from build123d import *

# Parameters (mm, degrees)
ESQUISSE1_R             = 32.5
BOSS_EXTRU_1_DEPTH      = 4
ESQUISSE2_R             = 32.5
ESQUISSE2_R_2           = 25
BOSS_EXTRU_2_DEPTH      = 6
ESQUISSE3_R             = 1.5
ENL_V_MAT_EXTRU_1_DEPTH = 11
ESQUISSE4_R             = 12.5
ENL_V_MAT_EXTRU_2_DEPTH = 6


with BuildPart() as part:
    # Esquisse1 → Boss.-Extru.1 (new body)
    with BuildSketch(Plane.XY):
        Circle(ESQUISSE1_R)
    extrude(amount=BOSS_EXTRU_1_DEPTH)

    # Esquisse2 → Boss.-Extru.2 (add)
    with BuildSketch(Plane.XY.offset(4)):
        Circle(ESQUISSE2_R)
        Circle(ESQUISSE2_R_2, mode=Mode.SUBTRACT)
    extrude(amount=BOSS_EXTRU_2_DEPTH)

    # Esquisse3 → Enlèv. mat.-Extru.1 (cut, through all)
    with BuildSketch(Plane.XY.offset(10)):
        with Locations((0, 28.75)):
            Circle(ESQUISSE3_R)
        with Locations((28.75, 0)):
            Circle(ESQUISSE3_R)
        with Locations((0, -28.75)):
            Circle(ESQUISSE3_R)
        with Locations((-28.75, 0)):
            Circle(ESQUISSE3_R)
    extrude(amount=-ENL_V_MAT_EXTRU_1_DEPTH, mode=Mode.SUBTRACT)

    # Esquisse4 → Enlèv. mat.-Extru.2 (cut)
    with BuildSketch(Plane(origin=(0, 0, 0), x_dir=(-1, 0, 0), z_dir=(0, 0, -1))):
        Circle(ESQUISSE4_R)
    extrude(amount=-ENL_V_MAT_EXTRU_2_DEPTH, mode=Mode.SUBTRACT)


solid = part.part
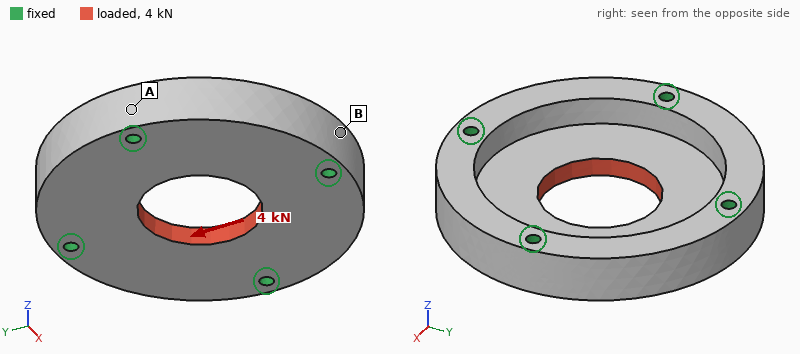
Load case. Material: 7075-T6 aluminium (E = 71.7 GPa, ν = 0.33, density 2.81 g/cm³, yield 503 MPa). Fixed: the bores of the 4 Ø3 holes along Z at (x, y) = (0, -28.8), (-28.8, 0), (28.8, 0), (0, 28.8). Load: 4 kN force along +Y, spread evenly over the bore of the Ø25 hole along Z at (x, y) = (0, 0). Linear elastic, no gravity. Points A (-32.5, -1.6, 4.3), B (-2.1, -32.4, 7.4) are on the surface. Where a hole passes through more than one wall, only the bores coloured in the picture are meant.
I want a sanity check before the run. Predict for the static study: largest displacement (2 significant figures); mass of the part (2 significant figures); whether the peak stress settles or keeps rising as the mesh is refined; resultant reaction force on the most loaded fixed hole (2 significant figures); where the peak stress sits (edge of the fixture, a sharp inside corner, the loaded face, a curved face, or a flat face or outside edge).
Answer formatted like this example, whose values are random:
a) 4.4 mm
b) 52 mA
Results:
a) 6.1 µm
b) 54 g
c) keeps rising
d) 1.1 kN
e) edge of the fixture
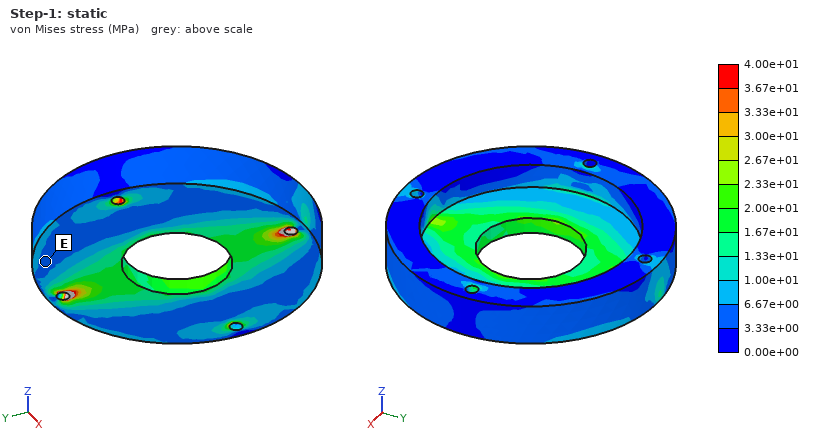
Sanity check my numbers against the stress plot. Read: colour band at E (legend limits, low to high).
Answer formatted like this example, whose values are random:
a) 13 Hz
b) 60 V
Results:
a) 3.33e+00 to 6.67e+00 MPa
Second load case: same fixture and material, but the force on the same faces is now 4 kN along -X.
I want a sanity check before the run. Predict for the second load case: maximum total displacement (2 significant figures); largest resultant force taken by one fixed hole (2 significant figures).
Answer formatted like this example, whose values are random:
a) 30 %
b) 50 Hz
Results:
a) 6.1 µm
b) 1.1 kN
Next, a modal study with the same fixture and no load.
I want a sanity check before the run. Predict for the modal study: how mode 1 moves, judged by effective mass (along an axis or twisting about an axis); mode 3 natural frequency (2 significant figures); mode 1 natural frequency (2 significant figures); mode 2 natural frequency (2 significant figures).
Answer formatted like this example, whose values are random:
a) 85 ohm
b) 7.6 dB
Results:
a) along Z
b) 18 kHz
c) 16 kHz
d) 18 kHz
